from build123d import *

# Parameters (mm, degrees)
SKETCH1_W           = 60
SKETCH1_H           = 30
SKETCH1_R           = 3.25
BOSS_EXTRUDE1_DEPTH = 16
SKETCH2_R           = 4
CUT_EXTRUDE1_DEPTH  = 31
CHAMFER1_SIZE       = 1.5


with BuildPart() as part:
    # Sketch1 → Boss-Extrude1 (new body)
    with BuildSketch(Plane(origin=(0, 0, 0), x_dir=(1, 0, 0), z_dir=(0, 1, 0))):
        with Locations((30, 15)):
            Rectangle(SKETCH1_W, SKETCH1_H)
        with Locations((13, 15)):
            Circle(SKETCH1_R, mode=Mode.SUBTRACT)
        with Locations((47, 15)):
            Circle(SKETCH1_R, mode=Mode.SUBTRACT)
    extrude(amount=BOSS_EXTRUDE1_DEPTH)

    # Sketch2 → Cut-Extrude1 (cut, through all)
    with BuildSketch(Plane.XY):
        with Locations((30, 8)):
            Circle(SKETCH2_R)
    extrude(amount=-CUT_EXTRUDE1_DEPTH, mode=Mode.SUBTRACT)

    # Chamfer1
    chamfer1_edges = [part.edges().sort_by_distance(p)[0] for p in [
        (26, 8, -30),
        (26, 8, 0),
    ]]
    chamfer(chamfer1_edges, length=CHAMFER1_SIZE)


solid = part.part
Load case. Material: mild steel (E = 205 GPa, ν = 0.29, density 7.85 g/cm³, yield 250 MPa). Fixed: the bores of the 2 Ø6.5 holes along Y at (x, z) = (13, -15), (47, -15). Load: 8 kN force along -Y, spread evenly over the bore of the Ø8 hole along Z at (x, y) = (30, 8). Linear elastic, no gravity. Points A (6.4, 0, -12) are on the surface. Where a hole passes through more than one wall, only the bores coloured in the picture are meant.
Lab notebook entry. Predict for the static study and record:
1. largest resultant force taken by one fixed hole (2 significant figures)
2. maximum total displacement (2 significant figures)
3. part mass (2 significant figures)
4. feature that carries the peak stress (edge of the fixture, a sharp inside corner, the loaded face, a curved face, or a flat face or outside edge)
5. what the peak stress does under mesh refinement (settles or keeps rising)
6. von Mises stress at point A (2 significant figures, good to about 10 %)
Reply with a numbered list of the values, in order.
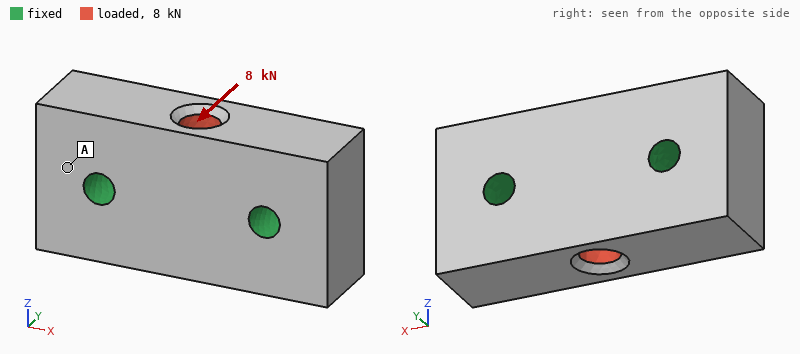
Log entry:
1. 4.0 kN
2. 3.2 µm
3. 210 g
4. edge of the fixture
5. keeps rising
6. 10.0 MPa
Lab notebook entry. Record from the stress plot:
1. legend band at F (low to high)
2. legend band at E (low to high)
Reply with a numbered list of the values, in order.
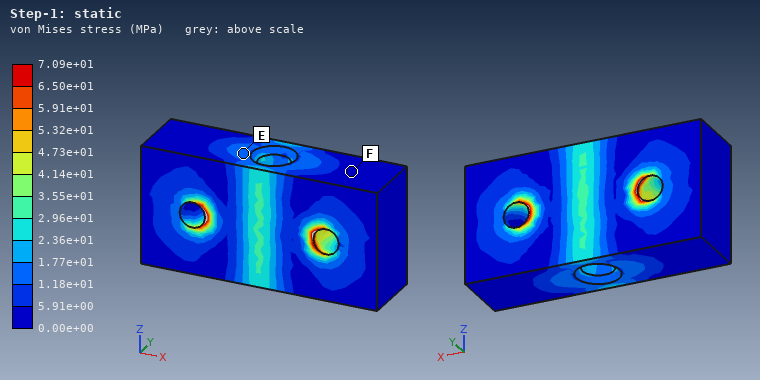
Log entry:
1. 0.00e+00 to 5.91e+00 MPa
2. 1.18e+01 to 1.77e+01 MPa
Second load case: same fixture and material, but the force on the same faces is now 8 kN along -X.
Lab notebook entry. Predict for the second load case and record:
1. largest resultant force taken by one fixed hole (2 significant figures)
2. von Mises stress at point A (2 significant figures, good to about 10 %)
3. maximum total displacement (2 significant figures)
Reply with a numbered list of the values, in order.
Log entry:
1. 4.0 kN
2. 4.5 MPa
3. 1.00 µm
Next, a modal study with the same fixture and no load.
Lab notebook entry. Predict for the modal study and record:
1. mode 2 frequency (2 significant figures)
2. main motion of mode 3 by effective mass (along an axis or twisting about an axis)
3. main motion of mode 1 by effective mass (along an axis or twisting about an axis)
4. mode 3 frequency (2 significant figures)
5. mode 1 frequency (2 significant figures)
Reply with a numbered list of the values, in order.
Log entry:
1. 31 kHz
2. twisting about Y
3. twisting about X
4. 33 kHz
5. 29 kHz
